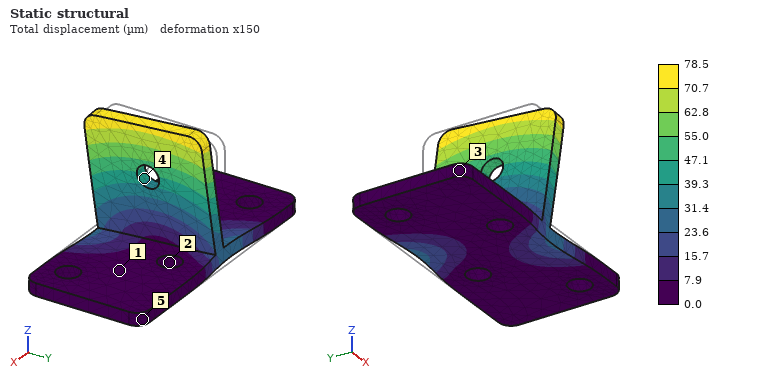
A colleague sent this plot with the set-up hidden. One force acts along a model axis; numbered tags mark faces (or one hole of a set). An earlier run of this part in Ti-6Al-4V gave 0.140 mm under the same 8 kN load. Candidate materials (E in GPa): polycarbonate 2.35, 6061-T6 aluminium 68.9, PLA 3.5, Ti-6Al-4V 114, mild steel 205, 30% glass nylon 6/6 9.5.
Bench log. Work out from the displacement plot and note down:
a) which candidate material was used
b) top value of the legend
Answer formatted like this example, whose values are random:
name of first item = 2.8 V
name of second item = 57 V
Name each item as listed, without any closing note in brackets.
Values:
which candidate material was used = mild steel
top value of the legend = 78.5 µm
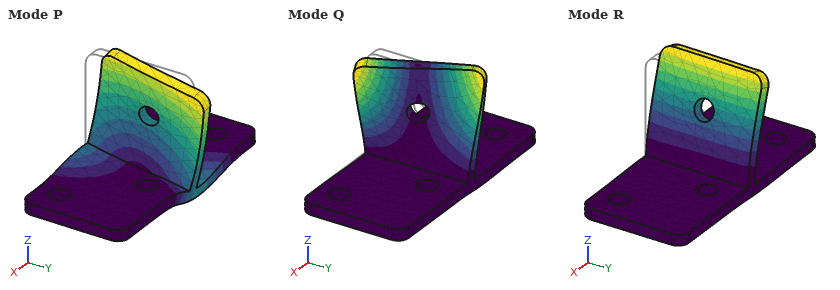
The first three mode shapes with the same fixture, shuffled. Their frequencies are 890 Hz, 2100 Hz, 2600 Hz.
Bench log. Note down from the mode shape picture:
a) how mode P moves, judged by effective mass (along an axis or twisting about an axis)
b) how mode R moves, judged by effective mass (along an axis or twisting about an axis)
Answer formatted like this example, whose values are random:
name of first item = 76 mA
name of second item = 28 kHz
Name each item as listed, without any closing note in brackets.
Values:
how mode P moves, judged by effective mass = along Y
how mode R moves, judged by effective mass = along X
